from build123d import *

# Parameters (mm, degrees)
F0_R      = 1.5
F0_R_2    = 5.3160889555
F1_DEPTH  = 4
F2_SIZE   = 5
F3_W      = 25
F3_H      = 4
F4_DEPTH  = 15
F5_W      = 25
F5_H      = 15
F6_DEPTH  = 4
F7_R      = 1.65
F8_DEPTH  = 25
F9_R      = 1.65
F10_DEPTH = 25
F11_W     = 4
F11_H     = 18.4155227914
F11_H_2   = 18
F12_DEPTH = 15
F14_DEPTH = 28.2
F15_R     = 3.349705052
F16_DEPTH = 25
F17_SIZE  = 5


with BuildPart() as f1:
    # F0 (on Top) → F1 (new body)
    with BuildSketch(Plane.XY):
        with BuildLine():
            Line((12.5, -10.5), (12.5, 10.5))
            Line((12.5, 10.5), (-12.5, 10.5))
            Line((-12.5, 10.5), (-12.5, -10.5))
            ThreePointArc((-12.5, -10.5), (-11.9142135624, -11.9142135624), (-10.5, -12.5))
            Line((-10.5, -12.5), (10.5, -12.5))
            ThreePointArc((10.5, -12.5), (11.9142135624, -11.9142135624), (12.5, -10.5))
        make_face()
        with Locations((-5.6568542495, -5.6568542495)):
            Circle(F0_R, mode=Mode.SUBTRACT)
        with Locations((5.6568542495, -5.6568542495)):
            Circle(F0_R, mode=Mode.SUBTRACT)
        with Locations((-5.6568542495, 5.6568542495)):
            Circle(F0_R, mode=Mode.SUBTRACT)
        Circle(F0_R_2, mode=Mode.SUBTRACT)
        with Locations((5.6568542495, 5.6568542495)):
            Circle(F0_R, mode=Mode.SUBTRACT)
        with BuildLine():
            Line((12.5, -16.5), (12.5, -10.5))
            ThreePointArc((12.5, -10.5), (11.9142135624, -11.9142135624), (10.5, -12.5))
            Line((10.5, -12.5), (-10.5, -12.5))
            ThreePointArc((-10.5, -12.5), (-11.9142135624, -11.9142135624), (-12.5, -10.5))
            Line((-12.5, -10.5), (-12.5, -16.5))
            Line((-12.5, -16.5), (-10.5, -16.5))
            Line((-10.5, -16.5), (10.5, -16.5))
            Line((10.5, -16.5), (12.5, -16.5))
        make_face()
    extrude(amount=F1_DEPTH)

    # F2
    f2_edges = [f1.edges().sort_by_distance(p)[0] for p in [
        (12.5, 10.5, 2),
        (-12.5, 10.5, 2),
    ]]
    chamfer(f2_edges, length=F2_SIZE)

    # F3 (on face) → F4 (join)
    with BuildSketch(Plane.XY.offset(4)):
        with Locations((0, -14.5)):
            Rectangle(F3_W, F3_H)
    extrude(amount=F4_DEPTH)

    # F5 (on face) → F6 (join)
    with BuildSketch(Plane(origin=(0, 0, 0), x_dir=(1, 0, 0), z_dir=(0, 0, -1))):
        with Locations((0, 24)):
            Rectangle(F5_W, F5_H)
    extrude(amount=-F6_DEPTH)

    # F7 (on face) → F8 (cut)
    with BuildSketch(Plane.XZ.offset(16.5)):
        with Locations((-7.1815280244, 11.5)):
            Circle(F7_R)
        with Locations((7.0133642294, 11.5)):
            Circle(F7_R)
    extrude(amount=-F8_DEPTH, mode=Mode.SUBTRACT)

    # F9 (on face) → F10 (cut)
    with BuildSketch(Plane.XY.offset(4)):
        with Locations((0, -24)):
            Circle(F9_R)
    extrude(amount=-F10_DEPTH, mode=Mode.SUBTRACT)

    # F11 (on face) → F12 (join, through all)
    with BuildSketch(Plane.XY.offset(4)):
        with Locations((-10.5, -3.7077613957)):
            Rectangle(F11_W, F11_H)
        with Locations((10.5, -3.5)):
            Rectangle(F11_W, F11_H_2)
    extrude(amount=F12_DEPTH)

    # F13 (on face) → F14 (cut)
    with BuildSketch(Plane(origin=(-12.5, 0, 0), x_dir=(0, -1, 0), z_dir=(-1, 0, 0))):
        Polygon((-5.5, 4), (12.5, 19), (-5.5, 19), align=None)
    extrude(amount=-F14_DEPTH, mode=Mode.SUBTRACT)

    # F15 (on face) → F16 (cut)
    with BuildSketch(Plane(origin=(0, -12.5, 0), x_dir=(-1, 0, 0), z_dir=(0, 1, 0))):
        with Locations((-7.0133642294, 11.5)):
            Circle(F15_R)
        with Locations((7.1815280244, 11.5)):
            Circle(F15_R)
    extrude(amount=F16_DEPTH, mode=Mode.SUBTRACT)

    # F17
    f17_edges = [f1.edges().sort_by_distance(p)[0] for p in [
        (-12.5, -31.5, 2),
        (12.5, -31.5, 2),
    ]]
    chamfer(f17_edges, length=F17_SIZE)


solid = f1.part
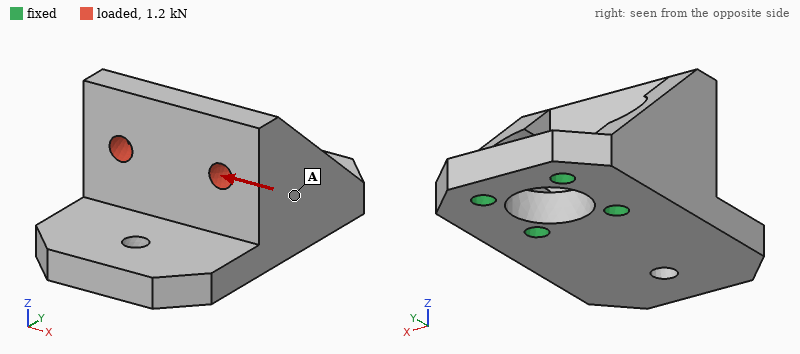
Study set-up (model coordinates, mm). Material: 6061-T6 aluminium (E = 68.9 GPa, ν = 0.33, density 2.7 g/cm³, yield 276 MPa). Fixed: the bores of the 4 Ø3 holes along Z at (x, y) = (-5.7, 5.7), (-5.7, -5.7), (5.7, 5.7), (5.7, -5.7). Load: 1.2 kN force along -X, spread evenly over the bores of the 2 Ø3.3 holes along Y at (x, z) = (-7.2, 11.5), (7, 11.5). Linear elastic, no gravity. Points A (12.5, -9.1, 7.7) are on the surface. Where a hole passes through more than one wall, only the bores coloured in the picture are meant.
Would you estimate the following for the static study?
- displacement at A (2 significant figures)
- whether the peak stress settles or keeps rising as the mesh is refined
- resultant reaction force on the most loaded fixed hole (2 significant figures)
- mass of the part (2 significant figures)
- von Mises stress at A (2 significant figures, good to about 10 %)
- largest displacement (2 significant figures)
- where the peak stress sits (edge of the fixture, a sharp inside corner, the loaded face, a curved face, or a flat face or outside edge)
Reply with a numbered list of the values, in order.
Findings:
1. 19 µm
2. keeps rising
3. 1.1 kN
4. 16 g
5. 17 MPa
6. 42 µm
7. edge of the fixture
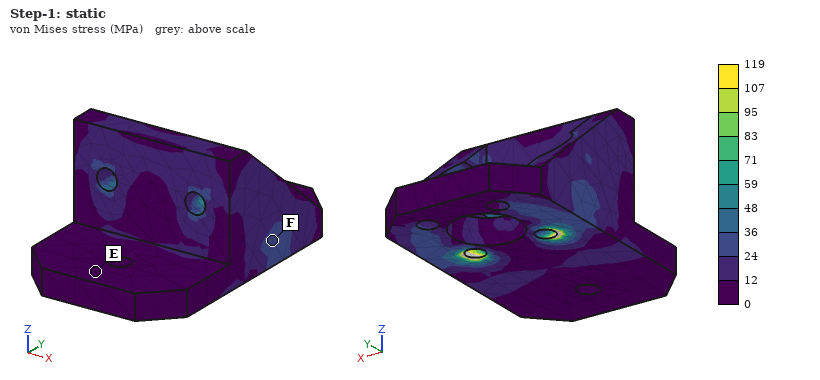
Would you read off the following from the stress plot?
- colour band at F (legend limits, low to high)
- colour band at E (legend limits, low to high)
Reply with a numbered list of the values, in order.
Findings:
1. 24 to 36 MPa
2. 0 to 12 MPa
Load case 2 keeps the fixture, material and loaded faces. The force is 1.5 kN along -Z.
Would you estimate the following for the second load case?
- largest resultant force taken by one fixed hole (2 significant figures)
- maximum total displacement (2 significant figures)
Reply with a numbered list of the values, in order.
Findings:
1. 1.1 kN
2. 58 µm
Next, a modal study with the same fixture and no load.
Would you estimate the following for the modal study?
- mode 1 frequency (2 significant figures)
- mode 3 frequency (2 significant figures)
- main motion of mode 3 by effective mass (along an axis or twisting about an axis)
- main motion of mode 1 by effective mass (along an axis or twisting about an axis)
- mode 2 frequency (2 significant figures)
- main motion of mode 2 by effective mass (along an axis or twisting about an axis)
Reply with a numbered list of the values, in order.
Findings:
1. 7300 Hz
2. 18 kHz
3. along X
4. along Z
5. 11 kHz
6. along X
